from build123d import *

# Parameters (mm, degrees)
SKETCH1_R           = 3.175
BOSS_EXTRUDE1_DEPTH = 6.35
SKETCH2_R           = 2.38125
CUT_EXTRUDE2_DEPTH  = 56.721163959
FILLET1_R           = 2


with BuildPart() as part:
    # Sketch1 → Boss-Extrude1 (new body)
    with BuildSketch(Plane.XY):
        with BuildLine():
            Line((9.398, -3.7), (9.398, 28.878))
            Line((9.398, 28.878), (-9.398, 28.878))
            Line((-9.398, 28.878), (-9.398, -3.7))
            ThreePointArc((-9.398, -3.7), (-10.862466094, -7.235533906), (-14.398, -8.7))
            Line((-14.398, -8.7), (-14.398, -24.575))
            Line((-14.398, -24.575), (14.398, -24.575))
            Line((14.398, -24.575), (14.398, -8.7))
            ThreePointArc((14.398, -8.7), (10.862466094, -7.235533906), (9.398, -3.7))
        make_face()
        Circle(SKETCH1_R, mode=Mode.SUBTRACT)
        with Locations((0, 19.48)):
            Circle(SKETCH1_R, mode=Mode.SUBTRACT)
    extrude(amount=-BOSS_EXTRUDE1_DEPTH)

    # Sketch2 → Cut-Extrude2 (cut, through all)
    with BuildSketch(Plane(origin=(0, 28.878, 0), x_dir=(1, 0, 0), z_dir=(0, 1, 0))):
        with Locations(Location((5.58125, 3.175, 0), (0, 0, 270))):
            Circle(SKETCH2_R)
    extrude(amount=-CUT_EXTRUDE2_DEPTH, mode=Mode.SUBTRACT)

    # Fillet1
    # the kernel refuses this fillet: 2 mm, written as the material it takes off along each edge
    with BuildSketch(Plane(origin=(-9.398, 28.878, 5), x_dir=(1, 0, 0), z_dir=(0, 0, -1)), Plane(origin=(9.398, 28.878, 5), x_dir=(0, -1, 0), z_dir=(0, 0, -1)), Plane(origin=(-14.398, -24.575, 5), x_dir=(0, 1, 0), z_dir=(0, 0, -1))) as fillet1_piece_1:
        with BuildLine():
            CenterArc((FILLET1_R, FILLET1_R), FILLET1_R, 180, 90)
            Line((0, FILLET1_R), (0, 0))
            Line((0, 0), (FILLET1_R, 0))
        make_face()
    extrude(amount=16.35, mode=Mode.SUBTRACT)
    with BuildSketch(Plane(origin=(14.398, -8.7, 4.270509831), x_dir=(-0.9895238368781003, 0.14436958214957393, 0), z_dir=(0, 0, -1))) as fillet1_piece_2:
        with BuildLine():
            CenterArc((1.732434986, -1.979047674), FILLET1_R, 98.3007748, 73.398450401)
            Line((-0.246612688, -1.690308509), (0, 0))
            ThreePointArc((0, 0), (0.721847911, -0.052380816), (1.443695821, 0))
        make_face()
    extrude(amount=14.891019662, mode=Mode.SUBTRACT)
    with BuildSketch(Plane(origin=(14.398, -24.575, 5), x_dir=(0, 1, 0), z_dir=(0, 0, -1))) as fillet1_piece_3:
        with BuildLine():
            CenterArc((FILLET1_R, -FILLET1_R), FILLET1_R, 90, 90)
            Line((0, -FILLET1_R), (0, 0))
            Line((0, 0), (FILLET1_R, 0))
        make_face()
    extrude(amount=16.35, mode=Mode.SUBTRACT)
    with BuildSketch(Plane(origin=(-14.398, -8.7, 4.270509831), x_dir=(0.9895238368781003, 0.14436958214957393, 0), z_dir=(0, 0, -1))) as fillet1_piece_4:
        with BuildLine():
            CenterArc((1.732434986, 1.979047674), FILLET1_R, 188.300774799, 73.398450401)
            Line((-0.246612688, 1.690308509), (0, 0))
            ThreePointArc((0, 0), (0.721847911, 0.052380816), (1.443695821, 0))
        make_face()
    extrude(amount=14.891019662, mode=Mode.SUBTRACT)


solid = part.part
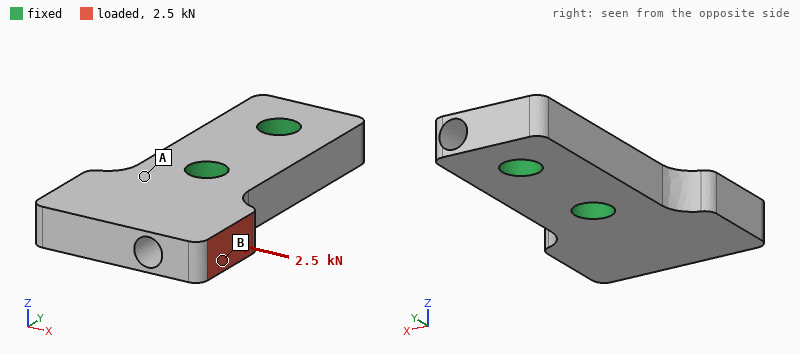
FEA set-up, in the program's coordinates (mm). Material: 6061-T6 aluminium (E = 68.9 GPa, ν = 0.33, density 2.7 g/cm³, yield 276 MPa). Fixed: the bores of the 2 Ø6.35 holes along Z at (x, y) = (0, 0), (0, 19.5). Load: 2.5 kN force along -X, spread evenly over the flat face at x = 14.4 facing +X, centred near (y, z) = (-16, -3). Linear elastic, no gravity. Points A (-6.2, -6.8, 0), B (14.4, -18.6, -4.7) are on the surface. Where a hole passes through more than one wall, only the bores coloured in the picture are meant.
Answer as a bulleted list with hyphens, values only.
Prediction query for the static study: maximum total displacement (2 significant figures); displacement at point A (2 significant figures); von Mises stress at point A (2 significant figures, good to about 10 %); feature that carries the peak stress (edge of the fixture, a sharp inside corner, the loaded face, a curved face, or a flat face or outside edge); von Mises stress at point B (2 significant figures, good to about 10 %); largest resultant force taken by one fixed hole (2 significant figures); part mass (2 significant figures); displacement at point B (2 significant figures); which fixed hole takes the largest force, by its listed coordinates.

- 87 µm
- 18 µm
- 56 MPa
- edge of the fixture
- 27 MPa
- 3.3 kN
- 16 g
- 76 µm
- (0, 0)
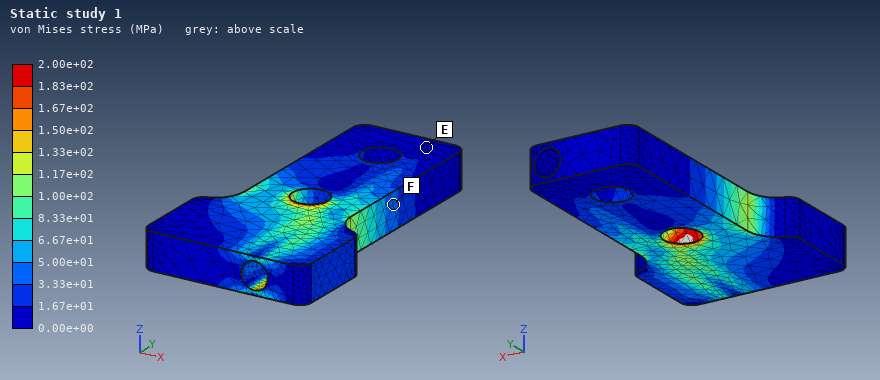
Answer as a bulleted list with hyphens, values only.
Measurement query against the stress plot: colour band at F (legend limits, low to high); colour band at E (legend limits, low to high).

- 3.33e+01 to 5.00e+01 MPa
- 0.00e+00 to 1.67e+01 MPa
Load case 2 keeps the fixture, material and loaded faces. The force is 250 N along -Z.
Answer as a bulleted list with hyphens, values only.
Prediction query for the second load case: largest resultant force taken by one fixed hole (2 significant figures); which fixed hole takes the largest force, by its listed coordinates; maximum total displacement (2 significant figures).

- 270 N
- (0, 0)
- 49 µm
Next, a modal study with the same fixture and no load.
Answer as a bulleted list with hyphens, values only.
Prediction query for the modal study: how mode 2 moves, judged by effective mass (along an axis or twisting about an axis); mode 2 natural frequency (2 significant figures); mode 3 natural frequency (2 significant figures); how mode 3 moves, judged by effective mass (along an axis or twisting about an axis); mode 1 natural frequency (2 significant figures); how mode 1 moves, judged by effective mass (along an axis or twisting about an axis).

- twisting about Y
- 11 kHz
- 12 kHz
- along X
- 7700 Hz
- along Z
